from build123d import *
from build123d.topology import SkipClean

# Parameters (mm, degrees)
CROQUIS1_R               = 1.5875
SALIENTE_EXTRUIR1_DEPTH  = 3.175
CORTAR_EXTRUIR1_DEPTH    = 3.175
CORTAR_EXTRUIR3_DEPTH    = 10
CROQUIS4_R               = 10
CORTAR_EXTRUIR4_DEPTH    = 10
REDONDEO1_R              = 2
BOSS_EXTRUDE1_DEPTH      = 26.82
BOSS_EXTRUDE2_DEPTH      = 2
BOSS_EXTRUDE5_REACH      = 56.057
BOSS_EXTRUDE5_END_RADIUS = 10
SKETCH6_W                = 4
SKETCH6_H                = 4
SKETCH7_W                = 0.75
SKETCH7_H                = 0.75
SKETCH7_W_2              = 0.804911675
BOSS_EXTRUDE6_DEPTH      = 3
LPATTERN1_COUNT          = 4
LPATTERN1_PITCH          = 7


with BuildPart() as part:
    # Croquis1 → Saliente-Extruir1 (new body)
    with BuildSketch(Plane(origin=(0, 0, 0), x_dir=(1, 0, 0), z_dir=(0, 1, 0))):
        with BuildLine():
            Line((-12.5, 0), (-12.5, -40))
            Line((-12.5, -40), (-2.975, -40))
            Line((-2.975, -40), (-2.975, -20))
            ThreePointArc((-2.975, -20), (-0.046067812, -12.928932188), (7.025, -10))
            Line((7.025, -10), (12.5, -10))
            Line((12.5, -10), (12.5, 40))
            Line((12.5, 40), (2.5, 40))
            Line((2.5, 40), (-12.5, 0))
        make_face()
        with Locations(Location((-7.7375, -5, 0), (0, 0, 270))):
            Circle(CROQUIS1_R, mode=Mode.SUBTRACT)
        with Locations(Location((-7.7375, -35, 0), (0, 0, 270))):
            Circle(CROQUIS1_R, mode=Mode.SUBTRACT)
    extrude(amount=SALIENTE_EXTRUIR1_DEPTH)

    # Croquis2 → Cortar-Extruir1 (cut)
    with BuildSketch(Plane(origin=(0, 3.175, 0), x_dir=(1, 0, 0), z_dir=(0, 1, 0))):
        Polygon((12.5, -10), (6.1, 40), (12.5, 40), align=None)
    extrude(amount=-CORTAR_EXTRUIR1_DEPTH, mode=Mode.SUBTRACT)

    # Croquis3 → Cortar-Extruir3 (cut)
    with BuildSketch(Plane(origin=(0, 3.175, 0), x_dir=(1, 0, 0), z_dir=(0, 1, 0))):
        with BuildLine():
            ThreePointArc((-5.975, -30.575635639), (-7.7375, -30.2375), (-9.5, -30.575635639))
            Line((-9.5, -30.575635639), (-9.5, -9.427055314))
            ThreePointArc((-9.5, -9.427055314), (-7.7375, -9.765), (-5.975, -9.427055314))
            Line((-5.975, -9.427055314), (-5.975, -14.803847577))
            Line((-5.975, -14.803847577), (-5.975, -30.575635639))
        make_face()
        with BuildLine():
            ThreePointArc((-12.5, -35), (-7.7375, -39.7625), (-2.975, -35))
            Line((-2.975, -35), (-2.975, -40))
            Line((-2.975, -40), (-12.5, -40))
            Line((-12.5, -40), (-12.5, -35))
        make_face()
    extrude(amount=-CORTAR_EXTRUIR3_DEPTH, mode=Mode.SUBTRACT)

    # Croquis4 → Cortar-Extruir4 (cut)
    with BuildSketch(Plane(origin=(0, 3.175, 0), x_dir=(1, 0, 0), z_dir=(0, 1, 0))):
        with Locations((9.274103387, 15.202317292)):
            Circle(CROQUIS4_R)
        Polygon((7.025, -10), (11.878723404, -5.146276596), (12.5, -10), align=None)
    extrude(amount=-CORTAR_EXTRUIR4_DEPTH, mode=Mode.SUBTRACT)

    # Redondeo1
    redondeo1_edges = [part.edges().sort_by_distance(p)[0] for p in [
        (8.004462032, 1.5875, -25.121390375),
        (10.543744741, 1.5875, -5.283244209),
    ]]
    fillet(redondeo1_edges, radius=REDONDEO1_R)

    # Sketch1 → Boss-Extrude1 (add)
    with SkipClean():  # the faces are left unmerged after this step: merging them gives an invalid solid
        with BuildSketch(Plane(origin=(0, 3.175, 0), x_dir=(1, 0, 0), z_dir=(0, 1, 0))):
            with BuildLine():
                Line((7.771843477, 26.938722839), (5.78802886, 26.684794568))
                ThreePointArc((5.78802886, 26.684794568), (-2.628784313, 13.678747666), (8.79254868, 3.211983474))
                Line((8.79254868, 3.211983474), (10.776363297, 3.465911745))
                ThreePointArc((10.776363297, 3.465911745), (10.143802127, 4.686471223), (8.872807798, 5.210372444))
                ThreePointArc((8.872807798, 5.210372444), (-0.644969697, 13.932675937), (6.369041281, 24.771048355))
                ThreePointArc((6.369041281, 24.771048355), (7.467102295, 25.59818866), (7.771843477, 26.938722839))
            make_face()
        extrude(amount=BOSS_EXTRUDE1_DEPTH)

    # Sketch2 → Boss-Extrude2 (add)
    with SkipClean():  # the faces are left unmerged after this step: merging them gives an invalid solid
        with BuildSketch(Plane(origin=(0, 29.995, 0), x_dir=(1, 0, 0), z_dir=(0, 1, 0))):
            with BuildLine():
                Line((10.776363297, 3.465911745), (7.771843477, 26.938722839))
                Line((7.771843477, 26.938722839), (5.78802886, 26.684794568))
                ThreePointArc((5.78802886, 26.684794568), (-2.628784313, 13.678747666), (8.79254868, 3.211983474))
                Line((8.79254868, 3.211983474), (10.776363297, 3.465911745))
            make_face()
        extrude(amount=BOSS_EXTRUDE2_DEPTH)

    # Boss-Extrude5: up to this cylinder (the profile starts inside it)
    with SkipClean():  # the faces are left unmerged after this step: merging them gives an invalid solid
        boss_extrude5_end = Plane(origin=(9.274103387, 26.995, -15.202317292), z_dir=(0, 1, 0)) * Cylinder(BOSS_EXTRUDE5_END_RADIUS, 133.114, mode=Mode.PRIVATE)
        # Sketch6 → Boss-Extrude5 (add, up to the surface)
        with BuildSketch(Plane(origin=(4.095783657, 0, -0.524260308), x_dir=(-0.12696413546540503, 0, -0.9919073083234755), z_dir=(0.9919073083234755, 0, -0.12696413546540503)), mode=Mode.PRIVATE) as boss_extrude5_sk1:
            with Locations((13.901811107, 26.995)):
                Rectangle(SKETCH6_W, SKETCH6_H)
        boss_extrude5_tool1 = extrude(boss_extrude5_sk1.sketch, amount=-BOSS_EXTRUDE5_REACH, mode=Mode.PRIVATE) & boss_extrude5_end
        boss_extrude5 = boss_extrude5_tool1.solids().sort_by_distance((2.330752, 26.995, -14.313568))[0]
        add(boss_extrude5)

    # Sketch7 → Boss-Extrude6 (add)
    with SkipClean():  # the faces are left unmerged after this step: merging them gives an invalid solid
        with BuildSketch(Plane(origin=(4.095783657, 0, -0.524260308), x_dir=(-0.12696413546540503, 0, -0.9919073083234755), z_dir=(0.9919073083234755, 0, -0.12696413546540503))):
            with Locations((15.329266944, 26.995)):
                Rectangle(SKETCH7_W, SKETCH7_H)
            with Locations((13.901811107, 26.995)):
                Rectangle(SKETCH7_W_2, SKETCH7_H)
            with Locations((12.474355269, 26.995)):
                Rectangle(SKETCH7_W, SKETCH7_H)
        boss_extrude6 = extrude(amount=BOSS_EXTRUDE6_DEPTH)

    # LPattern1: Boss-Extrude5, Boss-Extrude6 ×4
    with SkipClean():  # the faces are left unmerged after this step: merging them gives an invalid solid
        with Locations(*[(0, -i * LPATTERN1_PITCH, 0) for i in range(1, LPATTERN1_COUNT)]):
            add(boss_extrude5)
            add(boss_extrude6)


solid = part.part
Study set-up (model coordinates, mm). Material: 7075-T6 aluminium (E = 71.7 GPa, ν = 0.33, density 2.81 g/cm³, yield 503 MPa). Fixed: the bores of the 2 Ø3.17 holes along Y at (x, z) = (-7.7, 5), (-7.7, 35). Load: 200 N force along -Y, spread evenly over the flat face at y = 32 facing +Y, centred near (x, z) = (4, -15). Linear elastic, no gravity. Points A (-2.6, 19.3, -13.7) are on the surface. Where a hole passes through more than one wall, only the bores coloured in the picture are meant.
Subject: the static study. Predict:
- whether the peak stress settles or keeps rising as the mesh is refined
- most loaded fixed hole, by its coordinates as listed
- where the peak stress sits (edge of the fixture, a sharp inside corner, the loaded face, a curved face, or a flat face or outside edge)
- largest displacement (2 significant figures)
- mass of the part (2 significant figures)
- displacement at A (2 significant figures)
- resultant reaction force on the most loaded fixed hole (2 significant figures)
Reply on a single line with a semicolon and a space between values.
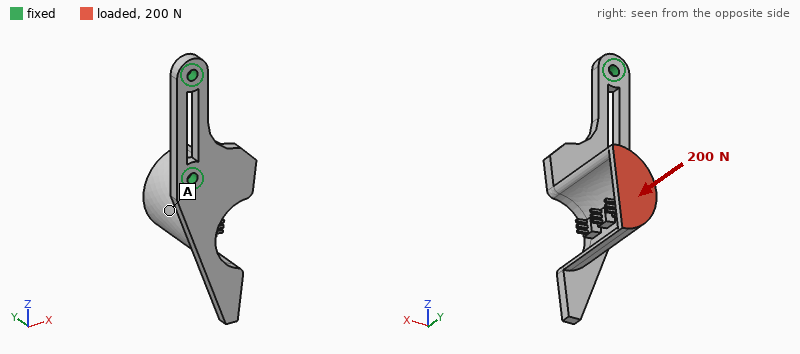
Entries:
keeps rising; (-7.7, 5); edge of the fixture; 0.65 mm; 14 g; 0.33 mm; 230 N
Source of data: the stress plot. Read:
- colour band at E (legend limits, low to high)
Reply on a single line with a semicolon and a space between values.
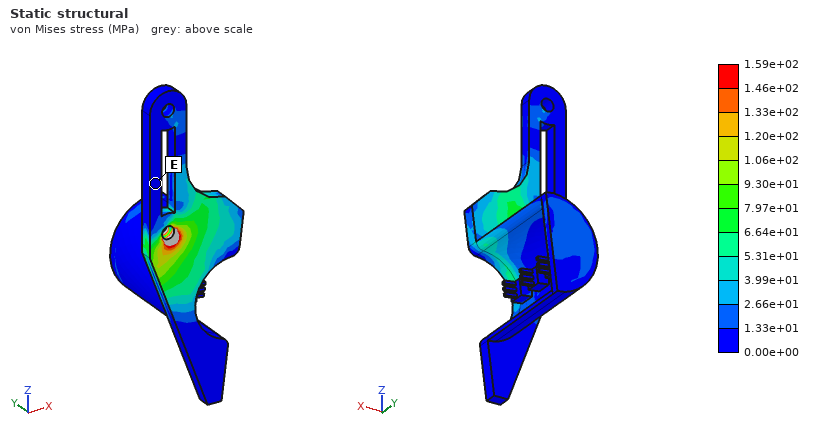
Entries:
0.00e+00 to 1.33e+01 MPa
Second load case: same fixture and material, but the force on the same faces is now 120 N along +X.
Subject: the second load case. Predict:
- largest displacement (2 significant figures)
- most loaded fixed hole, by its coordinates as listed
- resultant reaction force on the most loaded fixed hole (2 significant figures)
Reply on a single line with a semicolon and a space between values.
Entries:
0.63 mm; (-7.7, 5); 150 N
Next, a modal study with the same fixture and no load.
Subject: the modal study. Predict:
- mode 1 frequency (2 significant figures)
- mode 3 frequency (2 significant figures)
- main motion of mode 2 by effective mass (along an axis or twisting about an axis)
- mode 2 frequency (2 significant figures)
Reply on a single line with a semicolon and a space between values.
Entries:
930 Hz; 3300 Hz; along X; 1500 Hz
